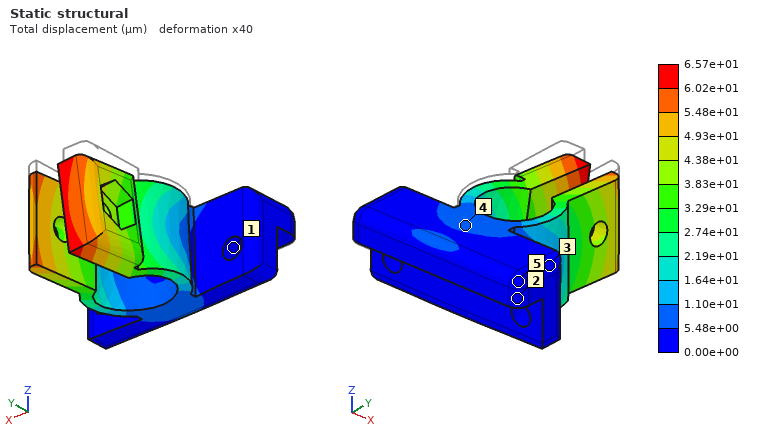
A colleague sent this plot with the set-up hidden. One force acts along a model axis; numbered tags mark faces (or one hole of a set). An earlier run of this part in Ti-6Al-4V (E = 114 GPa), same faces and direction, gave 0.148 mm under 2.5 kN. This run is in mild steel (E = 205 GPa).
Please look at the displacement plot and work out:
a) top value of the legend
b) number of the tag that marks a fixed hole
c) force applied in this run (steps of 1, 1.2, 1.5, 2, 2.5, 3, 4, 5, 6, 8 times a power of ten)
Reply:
6.57e+01 µm
1
2 kN
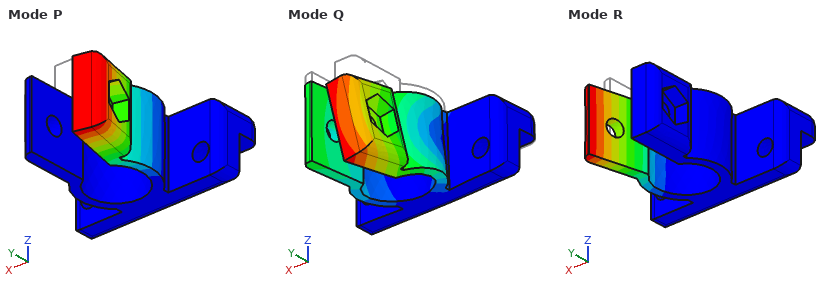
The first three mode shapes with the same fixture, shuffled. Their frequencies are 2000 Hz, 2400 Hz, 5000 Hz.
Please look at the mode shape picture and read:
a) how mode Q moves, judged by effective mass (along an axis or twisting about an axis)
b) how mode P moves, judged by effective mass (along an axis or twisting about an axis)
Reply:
along Z
along X
